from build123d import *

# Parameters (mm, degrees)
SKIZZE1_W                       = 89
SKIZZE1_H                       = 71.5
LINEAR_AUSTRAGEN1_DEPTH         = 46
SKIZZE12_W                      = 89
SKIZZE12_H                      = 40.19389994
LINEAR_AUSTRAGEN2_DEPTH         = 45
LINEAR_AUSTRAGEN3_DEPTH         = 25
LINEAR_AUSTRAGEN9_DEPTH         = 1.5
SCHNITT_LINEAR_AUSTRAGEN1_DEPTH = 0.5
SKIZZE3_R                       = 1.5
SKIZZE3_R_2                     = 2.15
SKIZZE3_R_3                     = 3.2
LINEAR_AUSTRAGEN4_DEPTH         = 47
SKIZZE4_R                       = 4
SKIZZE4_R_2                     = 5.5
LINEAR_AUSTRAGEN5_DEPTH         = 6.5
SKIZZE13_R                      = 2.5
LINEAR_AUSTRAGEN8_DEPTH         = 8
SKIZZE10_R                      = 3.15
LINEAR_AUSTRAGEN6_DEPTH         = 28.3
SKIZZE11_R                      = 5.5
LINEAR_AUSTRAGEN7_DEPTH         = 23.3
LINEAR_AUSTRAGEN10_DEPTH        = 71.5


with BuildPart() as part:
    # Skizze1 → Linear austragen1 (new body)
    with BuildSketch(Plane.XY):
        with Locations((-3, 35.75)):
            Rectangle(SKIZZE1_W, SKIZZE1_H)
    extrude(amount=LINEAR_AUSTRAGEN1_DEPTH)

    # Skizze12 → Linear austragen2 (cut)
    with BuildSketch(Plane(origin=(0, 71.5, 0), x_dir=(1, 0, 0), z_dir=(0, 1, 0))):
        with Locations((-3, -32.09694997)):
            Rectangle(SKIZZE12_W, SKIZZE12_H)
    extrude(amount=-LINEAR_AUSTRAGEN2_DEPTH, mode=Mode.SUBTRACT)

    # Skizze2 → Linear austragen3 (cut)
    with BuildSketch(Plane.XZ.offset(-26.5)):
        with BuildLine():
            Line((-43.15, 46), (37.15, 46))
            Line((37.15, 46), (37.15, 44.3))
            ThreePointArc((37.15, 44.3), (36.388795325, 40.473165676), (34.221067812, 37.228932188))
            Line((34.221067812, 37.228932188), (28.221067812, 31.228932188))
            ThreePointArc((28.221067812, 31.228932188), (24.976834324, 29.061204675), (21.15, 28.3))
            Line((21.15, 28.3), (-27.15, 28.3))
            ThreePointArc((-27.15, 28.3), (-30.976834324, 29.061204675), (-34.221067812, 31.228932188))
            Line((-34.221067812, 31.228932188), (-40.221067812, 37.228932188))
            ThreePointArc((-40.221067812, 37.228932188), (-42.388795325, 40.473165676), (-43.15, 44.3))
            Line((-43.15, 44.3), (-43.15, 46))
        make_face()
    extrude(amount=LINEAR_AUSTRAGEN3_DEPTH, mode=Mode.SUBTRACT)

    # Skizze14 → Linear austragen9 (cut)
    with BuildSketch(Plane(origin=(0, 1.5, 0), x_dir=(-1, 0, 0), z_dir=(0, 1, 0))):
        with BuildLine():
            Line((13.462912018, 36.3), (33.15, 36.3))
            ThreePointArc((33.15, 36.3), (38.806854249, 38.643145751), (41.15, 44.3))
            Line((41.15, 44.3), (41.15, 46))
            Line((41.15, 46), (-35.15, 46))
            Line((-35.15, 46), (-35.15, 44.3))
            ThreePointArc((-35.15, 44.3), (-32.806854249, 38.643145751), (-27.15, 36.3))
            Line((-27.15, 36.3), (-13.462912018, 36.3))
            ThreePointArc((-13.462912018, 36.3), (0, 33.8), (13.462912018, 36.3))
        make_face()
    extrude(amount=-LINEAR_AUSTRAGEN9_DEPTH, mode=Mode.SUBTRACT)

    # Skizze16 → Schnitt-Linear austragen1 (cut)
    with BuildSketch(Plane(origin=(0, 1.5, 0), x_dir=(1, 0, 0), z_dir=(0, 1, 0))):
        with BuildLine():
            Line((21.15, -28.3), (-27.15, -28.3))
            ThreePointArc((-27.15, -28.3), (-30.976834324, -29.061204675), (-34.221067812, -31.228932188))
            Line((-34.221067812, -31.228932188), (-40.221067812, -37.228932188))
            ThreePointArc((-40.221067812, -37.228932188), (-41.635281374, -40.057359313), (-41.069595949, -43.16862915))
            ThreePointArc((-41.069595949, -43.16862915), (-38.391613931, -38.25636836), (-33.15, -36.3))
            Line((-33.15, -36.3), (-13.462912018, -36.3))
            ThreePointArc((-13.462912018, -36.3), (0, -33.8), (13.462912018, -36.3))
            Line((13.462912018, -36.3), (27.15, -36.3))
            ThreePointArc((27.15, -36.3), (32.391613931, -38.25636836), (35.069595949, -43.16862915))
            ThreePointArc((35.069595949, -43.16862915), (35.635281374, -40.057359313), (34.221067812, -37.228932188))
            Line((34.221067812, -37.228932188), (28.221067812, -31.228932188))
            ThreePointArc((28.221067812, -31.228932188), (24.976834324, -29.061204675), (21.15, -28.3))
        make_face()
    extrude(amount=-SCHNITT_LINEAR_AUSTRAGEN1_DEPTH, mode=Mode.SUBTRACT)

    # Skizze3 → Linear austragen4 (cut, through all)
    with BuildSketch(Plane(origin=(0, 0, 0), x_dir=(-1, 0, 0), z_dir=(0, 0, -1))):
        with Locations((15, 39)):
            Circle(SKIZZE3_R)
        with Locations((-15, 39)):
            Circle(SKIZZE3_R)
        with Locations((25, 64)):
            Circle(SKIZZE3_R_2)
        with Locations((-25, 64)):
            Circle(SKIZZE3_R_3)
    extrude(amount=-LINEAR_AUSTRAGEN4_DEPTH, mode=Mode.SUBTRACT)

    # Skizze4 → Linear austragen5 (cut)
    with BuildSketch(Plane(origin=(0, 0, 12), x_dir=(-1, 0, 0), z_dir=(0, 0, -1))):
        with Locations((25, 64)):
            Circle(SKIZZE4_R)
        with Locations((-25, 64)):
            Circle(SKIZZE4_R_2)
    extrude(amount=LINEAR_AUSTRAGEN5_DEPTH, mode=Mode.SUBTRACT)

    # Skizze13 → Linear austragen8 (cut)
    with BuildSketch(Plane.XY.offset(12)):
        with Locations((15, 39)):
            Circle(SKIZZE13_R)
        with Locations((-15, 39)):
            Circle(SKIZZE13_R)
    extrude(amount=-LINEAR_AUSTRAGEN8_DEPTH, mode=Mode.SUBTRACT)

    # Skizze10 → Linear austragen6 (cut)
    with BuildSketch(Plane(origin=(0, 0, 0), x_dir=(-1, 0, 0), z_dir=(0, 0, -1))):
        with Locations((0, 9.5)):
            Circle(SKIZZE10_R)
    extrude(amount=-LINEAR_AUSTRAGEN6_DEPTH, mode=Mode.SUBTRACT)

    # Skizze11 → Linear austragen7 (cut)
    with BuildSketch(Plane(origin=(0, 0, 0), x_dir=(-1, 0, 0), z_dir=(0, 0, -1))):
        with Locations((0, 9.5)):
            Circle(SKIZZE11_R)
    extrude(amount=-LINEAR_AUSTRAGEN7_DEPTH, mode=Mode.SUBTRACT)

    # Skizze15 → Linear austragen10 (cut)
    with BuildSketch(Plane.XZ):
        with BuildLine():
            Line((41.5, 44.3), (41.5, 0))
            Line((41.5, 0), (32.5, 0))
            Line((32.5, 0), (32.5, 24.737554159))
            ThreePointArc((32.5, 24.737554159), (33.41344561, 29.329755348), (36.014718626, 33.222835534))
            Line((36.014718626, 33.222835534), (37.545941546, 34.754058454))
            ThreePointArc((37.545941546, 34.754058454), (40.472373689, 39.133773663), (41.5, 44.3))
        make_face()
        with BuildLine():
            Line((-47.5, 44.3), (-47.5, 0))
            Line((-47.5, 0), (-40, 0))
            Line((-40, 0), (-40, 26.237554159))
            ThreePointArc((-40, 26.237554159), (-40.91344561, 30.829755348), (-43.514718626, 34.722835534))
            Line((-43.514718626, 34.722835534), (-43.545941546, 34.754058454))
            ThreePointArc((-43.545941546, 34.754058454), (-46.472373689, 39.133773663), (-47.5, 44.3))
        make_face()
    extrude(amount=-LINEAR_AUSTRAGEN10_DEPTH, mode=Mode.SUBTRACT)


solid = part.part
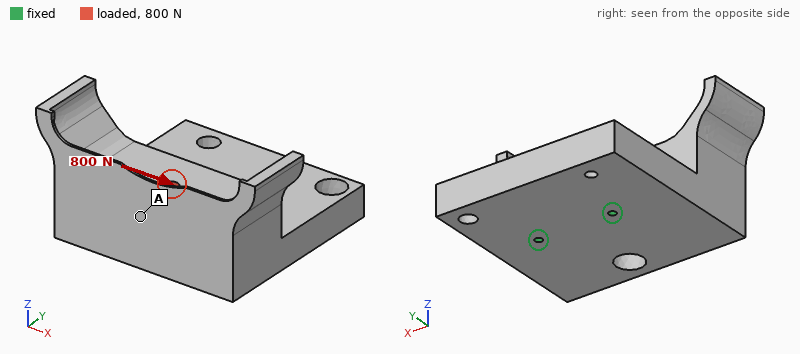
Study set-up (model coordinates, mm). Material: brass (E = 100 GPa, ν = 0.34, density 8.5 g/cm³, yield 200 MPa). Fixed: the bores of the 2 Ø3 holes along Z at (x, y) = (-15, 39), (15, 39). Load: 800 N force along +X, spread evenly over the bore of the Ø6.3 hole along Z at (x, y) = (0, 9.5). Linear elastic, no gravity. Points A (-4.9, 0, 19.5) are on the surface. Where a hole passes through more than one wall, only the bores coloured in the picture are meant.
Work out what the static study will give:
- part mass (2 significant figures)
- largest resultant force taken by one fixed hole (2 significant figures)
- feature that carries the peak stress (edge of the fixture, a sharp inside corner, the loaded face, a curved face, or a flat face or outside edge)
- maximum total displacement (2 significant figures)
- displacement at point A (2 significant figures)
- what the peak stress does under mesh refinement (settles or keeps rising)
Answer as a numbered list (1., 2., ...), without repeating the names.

1. 810 g
2. 1.1 kN
3. edge of the fixture
4. 12 µm
5. 5.6 µm
6. keeps rising
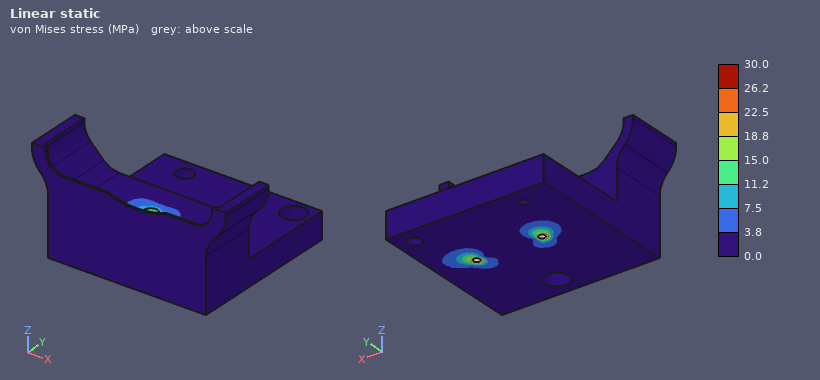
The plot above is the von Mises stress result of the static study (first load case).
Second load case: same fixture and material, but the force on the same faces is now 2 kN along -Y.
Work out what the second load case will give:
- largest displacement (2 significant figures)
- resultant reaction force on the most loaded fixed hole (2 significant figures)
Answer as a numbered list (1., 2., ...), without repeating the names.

1. 0.35 mm
2. 1.0 kN
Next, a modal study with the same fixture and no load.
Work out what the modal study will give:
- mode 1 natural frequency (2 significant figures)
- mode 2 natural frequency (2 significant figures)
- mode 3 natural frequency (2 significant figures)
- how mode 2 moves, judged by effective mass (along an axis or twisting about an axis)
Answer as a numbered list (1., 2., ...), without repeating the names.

1. 600 Hz
2. 2400 Hz
3. 2900 Hz
4. along X
